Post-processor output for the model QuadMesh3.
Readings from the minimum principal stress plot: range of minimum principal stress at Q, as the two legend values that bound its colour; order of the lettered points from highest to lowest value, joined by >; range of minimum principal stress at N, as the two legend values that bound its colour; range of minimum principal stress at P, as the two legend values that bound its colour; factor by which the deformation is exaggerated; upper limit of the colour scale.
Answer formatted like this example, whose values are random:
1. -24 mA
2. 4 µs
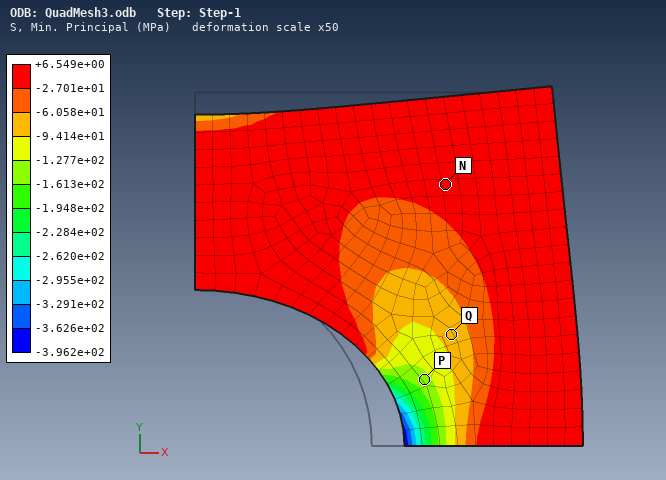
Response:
1. -9.414e+01 to -6.058e+01 MPa
2. N > Q > P
3. -2.701e+01 to +6.549e+00 MPa
4. -1.613e+02 to -1.277e+02 MPa
5. 50
6. +6.549e+00 MPa
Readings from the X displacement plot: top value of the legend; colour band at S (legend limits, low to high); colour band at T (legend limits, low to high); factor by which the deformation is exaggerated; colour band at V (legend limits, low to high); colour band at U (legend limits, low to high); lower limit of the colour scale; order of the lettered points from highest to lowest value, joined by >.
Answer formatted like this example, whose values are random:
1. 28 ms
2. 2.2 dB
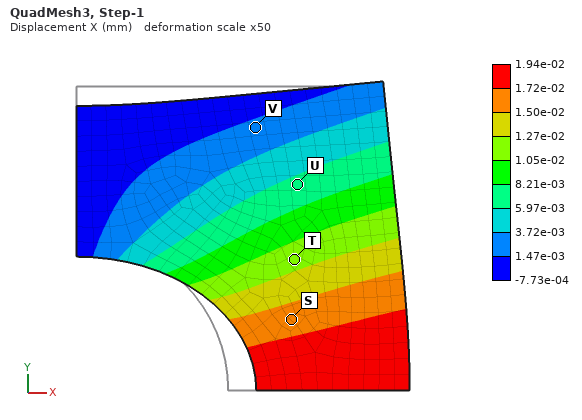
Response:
1. 1.94e-02 mm
2. 1.50e-02 to 1.72e-02 mm
3. 1.05e-02 to 1.27e-02 mm
4. 50
5. 1.47e-03 to 3.72e-03 mm
6. 5.97e-03 to 8.21e-03 mm
7. -7.73e-04 mm
8. S > T > U > V
